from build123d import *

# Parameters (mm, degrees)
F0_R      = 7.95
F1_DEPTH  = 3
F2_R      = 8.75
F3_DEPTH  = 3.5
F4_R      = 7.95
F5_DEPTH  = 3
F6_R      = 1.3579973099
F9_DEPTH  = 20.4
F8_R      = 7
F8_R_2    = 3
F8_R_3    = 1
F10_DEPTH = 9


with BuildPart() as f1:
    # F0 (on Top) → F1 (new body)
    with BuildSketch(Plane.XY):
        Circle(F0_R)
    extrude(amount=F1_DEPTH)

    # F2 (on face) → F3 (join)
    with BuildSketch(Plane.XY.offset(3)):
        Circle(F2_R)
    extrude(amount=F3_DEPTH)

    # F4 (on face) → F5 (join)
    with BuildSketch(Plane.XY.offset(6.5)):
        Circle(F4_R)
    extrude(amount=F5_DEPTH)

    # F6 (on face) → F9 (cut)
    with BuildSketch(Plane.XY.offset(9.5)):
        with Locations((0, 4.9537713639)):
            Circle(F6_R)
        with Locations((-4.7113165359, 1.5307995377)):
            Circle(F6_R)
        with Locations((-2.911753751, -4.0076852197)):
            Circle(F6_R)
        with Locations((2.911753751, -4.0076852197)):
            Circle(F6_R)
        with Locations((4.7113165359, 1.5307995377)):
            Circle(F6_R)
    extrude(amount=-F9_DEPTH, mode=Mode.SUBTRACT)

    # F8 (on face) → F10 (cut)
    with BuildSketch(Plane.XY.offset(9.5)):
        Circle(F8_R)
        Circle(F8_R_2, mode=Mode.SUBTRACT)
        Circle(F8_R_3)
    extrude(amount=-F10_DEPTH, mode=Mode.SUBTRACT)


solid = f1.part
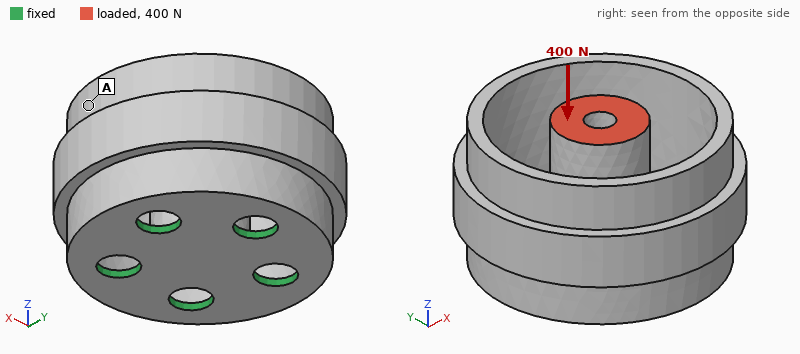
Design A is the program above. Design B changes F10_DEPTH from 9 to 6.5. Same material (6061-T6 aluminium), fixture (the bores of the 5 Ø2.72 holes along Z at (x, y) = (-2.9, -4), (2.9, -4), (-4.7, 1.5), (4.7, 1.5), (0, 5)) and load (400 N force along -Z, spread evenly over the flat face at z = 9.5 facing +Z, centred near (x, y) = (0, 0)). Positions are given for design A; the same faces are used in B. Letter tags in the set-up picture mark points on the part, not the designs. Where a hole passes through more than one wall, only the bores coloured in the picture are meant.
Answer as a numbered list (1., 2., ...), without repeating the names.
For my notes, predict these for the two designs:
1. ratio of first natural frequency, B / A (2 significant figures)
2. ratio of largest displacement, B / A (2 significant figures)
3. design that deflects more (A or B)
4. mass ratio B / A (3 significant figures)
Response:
1. 2.1
2. 0.29
3. A
4. 1.29
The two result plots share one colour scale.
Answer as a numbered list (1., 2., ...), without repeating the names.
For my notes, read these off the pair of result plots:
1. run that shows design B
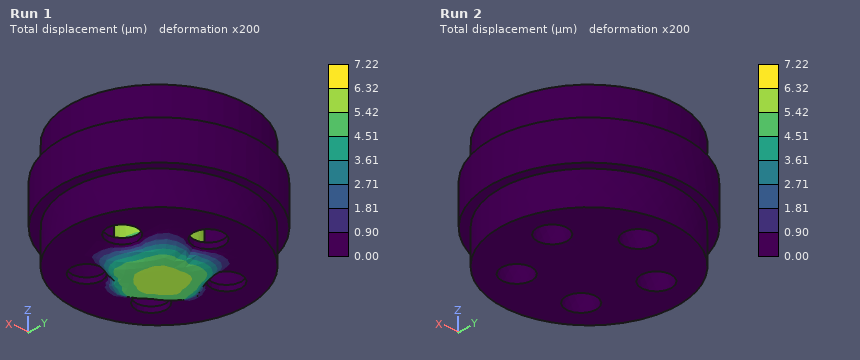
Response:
1. Run 2
